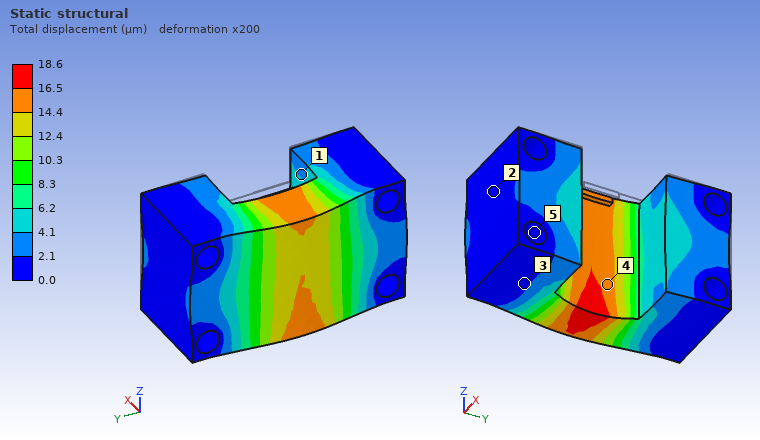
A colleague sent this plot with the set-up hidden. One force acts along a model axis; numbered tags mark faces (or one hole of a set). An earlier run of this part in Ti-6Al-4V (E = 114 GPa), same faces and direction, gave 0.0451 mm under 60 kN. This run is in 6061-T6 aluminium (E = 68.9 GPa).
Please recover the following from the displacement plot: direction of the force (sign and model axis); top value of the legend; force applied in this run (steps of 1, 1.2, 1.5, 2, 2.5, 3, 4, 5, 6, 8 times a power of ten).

-X
18.6 µm
15 kN
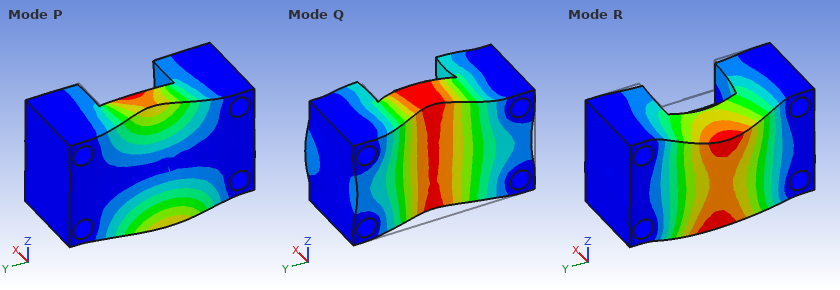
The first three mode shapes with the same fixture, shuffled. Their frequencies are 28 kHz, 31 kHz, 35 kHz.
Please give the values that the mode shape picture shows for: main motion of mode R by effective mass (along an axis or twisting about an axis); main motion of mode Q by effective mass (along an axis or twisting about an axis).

along Z
along X
